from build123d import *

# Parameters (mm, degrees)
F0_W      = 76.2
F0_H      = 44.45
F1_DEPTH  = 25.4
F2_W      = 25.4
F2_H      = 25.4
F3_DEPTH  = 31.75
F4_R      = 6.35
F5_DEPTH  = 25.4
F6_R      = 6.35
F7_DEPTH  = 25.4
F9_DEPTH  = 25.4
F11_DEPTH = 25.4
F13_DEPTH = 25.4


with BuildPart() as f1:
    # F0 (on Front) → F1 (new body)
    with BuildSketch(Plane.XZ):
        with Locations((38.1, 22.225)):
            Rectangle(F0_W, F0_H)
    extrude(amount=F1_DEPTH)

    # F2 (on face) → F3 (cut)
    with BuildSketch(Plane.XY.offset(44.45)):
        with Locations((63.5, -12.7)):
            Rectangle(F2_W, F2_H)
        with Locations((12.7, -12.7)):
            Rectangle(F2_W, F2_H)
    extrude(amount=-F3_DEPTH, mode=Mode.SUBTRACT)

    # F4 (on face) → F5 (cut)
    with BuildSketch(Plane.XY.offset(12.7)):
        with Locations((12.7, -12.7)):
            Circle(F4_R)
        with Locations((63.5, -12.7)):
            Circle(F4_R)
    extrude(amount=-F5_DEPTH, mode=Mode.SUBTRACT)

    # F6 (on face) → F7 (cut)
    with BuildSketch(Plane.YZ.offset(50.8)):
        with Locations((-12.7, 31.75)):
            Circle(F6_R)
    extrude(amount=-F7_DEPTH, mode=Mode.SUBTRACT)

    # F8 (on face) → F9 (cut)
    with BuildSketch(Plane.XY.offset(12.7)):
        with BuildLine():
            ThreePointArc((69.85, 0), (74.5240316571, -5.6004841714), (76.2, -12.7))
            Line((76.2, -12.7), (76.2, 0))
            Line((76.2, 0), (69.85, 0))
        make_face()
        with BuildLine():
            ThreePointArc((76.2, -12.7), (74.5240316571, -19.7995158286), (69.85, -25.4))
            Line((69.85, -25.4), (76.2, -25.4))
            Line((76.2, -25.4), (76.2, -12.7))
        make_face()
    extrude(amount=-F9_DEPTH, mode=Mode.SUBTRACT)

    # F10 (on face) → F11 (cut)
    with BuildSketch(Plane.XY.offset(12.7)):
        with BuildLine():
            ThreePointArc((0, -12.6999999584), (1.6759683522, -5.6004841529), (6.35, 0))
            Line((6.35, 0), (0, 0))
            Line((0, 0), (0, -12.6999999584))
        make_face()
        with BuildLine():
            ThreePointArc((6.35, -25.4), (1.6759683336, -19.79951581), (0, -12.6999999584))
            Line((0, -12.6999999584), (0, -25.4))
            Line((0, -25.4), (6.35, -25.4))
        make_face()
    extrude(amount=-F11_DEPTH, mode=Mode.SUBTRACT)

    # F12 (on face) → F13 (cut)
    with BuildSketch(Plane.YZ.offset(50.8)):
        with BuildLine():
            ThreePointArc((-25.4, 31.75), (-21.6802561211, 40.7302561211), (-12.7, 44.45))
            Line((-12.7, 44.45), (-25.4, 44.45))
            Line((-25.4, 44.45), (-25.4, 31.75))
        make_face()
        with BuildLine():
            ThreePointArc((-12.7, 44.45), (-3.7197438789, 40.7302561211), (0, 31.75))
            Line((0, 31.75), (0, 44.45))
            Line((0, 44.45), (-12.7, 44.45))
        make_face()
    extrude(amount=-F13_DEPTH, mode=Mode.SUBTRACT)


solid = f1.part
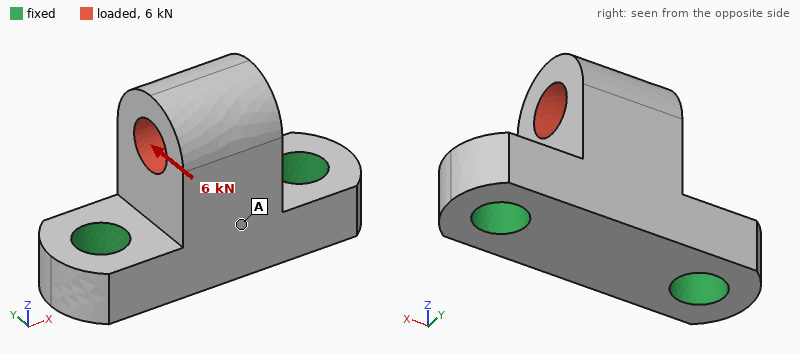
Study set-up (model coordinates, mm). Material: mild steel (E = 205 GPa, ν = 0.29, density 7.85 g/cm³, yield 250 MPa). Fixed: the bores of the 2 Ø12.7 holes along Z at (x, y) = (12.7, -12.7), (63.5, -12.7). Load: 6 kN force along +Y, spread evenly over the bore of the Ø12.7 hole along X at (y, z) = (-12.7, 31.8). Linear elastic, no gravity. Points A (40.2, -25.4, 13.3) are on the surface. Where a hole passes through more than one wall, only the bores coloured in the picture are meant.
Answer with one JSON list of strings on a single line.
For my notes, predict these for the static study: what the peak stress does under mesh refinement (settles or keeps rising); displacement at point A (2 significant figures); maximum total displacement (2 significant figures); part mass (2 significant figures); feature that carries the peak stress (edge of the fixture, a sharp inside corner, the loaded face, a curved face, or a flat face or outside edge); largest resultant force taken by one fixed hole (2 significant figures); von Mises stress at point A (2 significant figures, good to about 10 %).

["keeps rising", "14 µm", "44 µm", "280 g", "edge of the fixture", "3.0 kN", "26 MPa"]
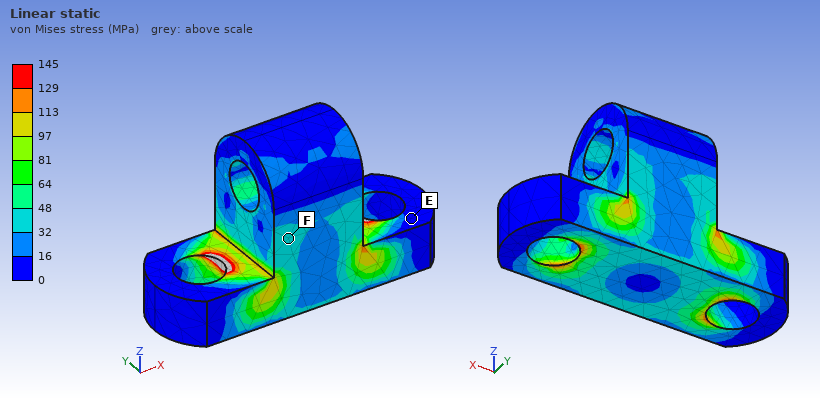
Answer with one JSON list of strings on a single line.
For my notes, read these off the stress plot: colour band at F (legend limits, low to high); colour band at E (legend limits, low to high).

["32 to 48 MPa", "0 to 16 MPa"]
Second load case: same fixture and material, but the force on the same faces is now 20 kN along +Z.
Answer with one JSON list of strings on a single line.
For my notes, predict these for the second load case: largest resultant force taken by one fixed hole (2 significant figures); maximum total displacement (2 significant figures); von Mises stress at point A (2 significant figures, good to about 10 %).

["10 kN", "15 µm", "20 MPa"]
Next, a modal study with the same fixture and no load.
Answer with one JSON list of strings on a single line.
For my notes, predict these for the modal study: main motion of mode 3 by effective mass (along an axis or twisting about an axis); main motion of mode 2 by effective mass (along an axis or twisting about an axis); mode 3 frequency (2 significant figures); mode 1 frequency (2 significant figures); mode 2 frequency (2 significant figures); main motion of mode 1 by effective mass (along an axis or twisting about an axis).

["along Z", "along X", "17 kHz", "7100 Hz", "12 kHz", "along Y"]
